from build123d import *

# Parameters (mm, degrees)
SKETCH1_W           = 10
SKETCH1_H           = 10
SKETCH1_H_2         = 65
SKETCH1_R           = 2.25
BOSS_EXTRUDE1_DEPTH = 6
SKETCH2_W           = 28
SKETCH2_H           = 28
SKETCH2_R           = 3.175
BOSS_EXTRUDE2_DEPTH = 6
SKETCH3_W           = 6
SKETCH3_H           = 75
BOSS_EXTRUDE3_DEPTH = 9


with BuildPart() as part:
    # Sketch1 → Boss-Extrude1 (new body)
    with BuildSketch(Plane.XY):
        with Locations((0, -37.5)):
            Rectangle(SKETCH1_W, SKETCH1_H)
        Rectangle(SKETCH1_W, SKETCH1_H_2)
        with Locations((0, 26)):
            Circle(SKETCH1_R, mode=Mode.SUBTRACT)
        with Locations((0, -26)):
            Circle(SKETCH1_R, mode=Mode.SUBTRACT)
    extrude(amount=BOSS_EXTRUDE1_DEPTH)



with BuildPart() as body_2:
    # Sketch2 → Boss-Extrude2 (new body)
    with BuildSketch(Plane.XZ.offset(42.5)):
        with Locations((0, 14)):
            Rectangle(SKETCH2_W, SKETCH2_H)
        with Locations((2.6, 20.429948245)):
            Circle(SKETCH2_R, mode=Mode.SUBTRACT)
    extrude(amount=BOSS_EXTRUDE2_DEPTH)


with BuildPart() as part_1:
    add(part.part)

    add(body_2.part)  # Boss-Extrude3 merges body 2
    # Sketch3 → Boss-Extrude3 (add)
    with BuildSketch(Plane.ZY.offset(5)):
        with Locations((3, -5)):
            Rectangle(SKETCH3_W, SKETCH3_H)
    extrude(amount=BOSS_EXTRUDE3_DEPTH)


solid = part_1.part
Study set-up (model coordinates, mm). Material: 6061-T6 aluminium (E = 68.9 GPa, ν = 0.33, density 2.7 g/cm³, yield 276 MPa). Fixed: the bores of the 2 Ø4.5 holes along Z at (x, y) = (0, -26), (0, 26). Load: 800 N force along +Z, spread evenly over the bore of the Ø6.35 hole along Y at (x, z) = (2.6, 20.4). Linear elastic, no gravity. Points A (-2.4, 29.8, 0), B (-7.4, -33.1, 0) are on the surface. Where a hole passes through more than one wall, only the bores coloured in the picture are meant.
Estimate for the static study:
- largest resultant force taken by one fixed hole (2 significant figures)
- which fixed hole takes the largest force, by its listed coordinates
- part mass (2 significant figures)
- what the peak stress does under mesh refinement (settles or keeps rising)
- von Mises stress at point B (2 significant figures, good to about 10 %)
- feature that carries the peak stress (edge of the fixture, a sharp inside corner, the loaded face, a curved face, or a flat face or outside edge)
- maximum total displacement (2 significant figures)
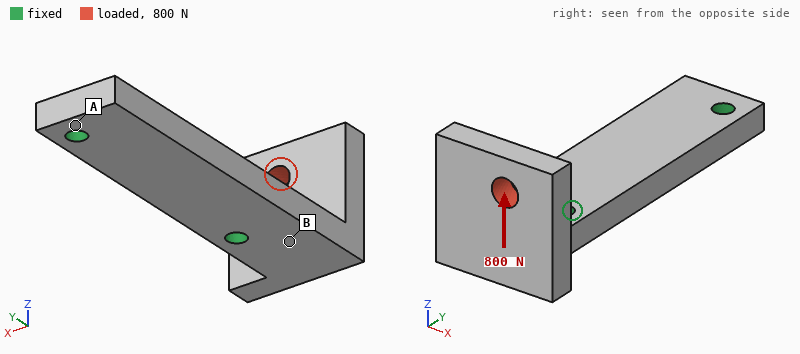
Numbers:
830 N
(0, -26)
35 g
keeps rising
72 MPa
edge of the fixture
0.23 mm
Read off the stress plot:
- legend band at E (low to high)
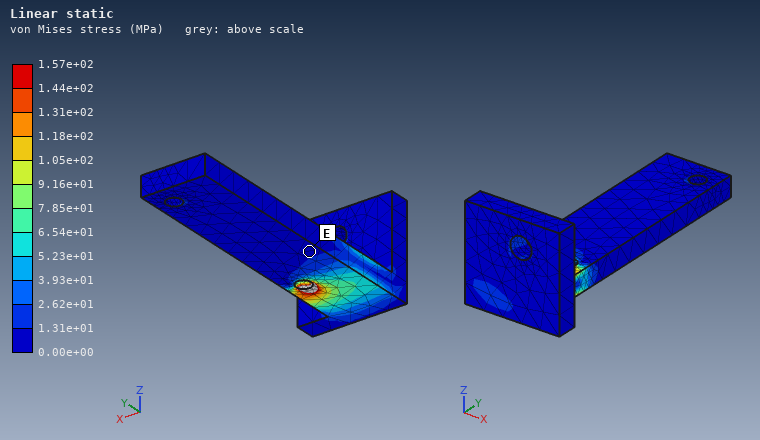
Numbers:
0.00e+00 to 1.31e+01 MPa
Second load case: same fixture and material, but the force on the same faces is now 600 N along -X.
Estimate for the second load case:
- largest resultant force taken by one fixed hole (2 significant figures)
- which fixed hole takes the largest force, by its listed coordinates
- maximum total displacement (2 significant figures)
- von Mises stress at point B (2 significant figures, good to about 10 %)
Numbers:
800 N
(0, -26)
0.21 mm
57 MPa
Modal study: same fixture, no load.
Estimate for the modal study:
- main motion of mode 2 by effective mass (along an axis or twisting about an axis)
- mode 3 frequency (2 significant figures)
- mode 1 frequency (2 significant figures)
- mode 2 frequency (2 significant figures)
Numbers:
along X
7900 Hz
2800 Hz
3500 Hz
